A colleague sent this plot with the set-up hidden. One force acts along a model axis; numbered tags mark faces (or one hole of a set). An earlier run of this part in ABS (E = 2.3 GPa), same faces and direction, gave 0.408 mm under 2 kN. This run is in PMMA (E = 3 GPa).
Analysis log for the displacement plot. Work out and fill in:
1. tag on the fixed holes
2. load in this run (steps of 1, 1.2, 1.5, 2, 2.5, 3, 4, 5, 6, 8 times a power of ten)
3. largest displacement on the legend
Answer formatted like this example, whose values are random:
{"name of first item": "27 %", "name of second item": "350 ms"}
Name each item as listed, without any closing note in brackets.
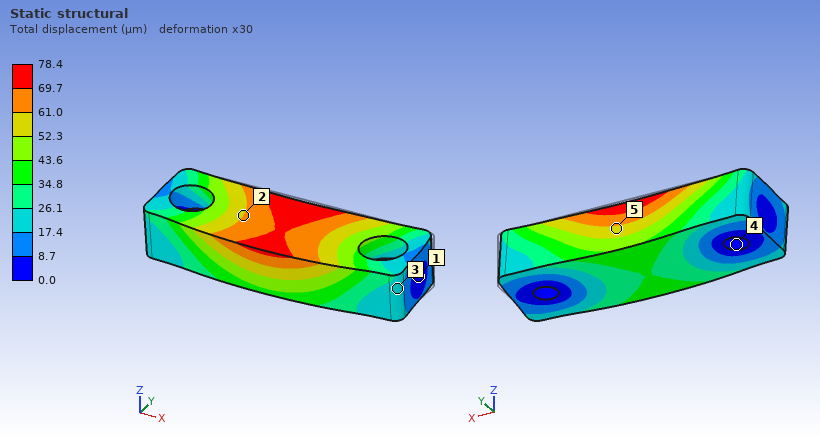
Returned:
{"tag on the fixed holes": "4", "load in this run": "500 N", "largest displacement on the legend": "78.4 µm"}
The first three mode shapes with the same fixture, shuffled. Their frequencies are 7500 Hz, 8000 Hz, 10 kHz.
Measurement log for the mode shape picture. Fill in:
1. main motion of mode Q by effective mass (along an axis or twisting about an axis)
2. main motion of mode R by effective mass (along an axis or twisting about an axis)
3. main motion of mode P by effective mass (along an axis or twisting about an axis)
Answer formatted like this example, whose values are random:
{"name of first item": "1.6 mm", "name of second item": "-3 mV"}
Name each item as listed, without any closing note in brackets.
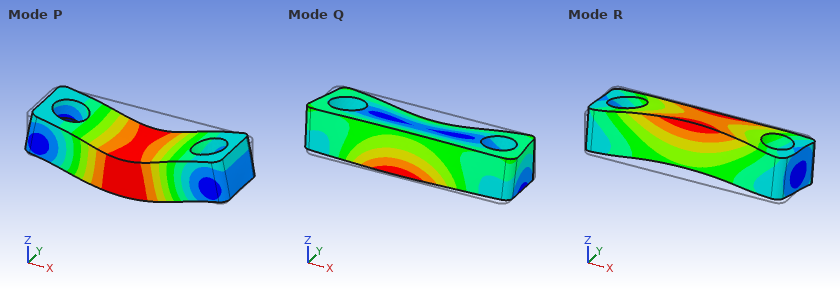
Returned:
{"main motion of mode Q by effective mass": "along Y", "main motion of mode R by effective mass": "along Y", "main motion of mode P by effective mass": "along Z"}
